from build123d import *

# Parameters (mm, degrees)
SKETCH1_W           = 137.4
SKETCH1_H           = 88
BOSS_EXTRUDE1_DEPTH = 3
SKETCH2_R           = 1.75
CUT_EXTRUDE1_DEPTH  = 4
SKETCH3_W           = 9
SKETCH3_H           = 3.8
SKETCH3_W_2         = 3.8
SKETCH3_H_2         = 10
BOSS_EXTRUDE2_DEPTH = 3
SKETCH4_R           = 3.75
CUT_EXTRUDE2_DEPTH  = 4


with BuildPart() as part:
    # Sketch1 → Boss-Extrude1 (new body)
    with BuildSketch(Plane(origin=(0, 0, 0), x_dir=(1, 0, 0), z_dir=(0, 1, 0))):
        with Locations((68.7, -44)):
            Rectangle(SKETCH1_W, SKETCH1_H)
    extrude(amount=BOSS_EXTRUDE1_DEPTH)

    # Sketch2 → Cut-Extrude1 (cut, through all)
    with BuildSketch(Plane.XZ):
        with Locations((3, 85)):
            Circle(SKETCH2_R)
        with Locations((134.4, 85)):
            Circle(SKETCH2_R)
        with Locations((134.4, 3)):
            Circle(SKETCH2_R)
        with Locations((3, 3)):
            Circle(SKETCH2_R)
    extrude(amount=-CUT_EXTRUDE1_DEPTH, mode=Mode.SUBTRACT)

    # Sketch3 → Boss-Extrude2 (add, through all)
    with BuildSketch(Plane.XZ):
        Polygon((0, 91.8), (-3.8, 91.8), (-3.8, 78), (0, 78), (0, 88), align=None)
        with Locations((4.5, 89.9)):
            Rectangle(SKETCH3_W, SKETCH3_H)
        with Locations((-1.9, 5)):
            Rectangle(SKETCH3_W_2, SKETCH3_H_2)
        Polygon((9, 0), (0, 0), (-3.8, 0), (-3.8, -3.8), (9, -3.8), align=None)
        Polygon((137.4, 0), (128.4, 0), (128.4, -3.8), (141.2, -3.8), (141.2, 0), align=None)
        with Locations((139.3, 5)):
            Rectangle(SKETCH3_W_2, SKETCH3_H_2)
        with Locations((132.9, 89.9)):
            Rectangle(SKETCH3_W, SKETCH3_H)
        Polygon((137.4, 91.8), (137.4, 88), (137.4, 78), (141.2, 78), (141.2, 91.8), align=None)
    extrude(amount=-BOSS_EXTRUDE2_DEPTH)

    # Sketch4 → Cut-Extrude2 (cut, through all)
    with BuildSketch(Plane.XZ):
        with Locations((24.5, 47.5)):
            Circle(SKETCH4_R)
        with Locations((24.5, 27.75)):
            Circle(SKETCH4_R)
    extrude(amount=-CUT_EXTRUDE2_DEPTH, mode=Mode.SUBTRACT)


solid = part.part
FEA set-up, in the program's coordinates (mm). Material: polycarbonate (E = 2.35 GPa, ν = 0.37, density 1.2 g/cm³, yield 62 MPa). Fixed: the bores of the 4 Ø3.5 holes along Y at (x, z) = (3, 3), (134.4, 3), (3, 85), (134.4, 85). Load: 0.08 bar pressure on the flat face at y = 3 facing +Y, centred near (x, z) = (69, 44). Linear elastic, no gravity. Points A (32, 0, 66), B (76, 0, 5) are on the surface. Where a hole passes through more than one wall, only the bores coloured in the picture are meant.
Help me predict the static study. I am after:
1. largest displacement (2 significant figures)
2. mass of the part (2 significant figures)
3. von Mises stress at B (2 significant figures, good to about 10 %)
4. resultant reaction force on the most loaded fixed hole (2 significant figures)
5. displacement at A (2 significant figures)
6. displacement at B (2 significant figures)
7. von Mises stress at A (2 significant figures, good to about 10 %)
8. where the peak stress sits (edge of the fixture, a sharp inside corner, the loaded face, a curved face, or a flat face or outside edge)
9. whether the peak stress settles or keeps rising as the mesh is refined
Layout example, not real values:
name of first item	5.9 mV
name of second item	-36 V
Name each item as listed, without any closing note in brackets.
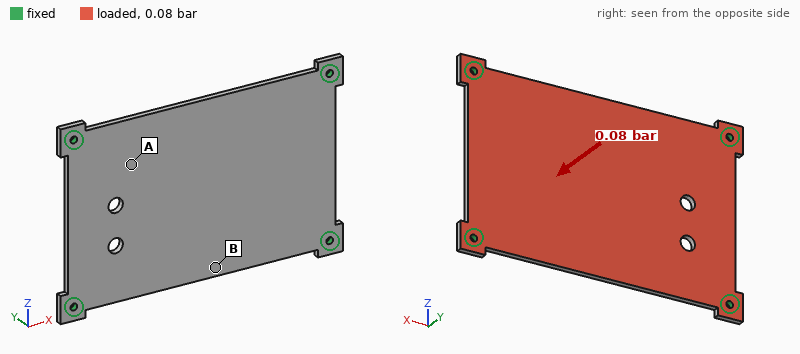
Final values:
largest displacement	2.0 mm
mass of the part	44 g
von Mises stress at B	5.4 MPa
resultant reaction force on the most loaded fixed hole	25 N
displacement at A	1.2 mm
displacement at B	1.9 mm
von Mises stress at A	2.2 MPa
where the peak stress sits	edge of the fixture
whether the peak stress settles or keeps rising as the mesh is refined	keeps rising
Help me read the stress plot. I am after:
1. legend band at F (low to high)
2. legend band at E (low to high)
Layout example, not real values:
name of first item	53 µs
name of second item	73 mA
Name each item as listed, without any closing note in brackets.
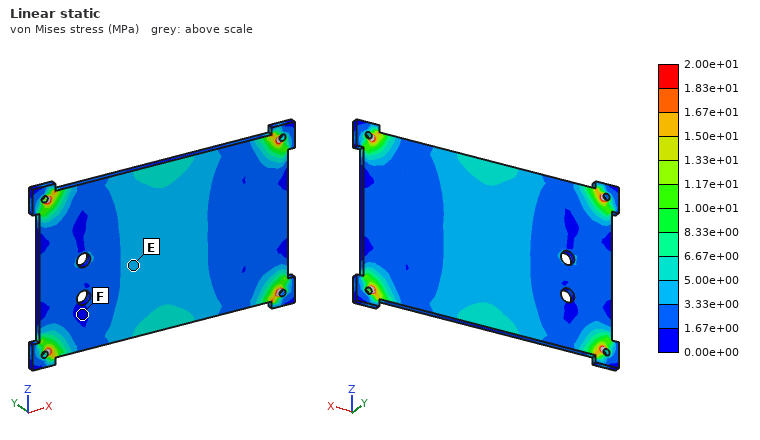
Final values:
legend band at F	0.00e+00 to 1.67e+00 MPa
legend band at E	3.33e+00 to 5.00e+00 MPa
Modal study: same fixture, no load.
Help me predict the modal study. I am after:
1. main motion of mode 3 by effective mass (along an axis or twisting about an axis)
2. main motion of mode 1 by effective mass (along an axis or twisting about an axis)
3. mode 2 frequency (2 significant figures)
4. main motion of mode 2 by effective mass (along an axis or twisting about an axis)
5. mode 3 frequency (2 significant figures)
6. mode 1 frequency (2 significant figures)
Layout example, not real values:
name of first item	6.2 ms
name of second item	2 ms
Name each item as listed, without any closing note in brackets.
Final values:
main motion of mode 3 by effective mass	twisting about Z
main motion of mode 1 by effective mass	along Y
mode 2 frequency	340 Hz
main motion of mode 2 by effective mass	twisting about X
mode 3 frequency	500 Hz
mode 1 frequency	190 Hz
